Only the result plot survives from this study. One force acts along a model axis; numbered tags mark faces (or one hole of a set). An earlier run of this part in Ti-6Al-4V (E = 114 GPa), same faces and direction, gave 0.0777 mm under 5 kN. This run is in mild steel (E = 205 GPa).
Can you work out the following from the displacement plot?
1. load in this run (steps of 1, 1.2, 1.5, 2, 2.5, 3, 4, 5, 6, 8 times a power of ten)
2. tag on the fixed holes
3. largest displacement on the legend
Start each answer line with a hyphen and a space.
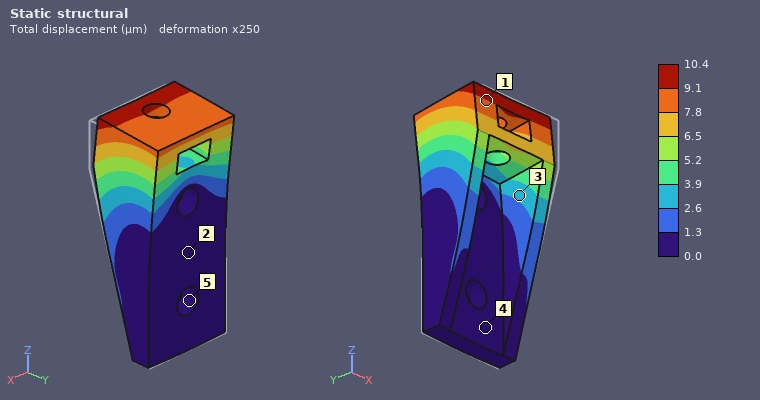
- 1.2 kN
- 5
- 10.4 µm
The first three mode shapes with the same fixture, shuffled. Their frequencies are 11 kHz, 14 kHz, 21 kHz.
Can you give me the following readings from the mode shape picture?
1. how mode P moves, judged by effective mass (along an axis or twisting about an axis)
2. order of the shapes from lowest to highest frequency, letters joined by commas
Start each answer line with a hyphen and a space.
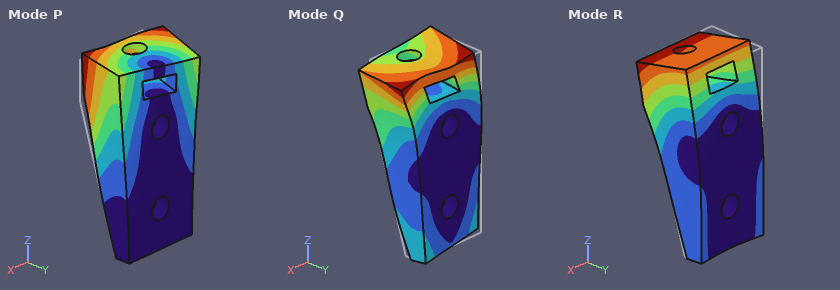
- along X
- P, R, Q
